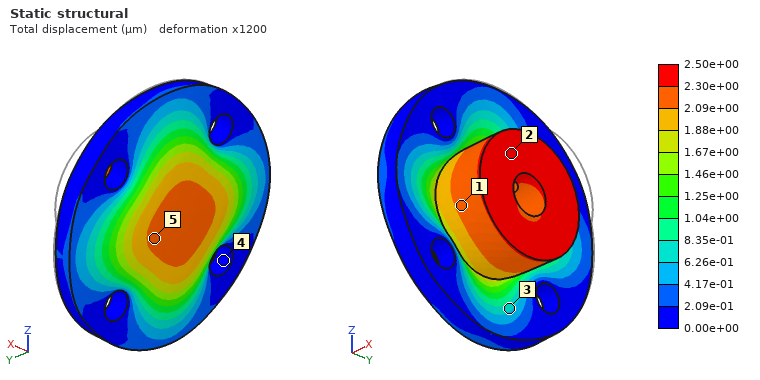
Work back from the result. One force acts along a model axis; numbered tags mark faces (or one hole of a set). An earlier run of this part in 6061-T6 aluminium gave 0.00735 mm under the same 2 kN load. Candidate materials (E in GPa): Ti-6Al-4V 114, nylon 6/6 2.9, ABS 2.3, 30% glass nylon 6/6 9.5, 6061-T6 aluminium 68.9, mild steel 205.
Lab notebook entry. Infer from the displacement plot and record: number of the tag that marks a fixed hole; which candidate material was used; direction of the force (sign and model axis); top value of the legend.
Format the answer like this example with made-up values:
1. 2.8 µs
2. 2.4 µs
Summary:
1. 4
2. mild steel
3. -X
4. 2.50e+00 µm
